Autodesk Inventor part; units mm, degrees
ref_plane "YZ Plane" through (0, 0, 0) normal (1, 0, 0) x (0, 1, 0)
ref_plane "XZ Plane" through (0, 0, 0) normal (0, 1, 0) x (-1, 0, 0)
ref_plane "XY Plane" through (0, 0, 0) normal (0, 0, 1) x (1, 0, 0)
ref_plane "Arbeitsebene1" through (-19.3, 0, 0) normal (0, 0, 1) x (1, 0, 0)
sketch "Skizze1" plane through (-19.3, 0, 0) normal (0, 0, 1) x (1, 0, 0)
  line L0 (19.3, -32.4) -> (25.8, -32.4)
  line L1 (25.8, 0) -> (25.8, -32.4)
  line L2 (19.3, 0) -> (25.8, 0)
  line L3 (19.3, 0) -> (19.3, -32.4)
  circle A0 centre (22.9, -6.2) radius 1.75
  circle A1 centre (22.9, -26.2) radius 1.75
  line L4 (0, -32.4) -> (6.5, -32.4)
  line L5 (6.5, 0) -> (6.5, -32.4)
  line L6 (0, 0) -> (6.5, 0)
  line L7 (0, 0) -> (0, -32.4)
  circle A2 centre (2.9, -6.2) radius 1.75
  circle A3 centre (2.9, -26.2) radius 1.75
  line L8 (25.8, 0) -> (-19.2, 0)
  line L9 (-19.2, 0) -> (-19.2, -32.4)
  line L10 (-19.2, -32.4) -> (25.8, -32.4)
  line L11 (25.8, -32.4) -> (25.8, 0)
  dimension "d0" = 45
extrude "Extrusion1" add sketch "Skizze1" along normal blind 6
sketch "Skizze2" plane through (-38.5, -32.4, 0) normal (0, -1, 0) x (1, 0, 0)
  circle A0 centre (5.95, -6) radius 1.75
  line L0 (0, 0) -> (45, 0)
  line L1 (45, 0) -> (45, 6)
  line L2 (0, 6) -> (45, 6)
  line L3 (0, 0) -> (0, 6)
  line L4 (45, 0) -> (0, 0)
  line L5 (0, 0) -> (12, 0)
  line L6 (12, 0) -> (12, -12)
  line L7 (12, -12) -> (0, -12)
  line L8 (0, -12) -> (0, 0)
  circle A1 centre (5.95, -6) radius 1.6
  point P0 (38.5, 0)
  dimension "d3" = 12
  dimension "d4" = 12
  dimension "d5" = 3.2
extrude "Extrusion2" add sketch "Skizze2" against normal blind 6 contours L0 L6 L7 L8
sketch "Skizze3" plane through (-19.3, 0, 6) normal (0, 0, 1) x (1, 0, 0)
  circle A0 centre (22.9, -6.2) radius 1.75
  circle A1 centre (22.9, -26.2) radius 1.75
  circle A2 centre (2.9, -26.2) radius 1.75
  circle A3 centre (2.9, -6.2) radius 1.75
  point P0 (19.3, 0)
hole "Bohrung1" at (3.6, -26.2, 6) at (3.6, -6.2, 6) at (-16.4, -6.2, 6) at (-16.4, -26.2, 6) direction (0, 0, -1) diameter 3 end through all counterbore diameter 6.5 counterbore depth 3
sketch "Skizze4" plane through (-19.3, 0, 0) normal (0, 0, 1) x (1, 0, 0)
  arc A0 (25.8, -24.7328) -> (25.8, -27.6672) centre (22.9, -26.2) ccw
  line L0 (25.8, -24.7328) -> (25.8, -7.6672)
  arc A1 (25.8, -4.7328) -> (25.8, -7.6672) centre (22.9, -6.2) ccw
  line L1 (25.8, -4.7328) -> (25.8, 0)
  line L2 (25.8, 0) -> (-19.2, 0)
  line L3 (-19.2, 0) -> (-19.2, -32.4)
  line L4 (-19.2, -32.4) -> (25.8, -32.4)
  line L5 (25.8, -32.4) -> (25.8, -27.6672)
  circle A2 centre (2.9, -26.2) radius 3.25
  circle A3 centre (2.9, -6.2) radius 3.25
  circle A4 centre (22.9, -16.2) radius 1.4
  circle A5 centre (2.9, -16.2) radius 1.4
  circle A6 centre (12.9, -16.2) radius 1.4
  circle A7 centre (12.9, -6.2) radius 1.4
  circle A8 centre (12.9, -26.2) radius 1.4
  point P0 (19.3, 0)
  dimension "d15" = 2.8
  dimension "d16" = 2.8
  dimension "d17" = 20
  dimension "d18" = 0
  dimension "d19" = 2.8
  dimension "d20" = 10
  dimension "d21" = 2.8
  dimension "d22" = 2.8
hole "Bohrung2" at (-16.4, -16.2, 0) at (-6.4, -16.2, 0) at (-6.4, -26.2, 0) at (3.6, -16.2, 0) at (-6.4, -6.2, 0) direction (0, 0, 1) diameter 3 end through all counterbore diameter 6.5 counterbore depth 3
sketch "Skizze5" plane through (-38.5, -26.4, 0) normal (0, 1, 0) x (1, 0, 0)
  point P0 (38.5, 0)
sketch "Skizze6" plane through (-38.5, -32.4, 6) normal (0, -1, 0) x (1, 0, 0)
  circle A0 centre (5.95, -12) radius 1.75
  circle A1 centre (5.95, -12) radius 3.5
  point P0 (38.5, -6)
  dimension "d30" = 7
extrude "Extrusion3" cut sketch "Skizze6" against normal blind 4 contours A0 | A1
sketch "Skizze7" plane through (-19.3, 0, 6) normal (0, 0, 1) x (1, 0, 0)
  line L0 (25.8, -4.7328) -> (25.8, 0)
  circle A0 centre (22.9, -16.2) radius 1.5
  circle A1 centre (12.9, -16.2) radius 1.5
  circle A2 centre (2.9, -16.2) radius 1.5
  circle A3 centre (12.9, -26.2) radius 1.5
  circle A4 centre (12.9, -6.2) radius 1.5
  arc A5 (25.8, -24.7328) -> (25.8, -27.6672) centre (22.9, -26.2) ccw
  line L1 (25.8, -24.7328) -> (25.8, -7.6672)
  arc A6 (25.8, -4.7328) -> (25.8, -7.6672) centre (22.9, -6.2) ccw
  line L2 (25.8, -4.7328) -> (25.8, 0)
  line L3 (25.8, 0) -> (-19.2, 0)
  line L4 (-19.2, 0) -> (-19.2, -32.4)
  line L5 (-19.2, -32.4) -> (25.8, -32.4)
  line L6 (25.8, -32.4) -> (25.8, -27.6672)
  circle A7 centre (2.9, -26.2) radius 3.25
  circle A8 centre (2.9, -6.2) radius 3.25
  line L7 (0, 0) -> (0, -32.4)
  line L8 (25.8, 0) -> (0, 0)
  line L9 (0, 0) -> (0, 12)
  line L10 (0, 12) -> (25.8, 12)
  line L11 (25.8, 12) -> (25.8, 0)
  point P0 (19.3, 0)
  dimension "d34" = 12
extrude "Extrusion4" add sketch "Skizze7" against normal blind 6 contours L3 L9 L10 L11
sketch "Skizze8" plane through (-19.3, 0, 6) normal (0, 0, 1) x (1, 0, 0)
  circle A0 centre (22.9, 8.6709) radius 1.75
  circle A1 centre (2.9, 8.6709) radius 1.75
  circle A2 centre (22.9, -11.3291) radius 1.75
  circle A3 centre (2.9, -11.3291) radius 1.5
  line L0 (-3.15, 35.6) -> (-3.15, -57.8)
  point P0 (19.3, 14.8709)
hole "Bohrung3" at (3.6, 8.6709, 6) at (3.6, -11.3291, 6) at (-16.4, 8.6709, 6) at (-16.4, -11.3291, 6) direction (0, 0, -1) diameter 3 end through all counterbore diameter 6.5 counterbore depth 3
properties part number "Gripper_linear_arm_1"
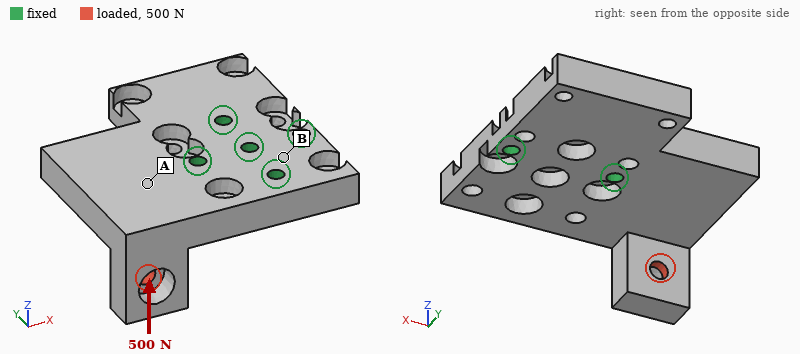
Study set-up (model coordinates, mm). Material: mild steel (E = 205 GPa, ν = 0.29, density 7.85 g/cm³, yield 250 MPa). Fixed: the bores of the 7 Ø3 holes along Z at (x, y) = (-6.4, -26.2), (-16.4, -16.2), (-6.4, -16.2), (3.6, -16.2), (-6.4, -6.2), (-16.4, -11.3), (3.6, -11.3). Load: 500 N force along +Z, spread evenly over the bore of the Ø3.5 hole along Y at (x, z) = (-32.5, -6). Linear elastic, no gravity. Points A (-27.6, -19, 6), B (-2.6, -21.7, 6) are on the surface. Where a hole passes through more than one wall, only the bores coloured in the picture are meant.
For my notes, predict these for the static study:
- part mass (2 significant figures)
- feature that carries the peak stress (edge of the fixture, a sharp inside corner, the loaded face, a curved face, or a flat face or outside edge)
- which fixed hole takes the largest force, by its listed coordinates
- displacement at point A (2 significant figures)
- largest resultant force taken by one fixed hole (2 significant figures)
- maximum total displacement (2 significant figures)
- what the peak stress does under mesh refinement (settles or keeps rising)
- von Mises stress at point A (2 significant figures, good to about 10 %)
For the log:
76 g
edge of the fixture
(-16.4, -16.2)
11 µm
1.2 kN
41 µm
keeps rising
26 MPa
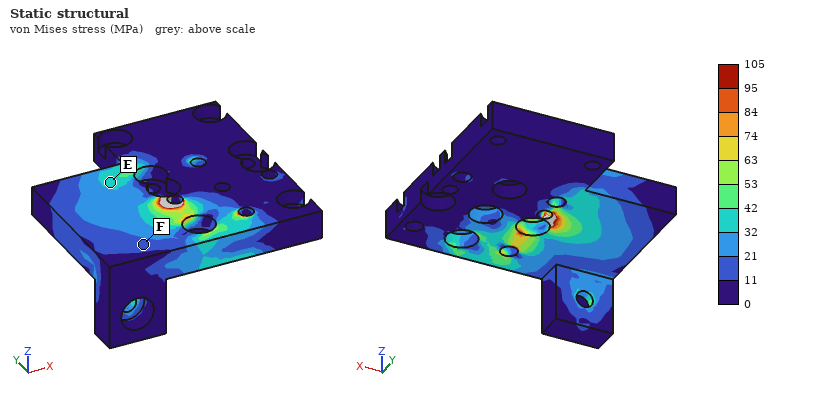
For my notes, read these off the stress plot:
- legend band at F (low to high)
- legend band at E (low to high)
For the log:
11 to 21 MPa
32 to 42 MPa
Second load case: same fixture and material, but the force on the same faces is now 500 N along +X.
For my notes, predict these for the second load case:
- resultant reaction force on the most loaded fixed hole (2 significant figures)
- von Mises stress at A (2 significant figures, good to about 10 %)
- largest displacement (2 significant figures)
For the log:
400 N
21 MPa
28 µm
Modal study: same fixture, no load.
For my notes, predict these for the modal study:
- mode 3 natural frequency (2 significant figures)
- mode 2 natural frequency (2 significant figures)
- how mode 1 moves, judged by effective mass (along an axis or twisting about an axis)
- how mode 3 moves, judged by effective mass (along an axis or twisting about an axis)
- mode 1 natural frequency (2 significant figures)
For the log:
10 kHz
8500 Hz
along Z
along Z
5200 Hz
